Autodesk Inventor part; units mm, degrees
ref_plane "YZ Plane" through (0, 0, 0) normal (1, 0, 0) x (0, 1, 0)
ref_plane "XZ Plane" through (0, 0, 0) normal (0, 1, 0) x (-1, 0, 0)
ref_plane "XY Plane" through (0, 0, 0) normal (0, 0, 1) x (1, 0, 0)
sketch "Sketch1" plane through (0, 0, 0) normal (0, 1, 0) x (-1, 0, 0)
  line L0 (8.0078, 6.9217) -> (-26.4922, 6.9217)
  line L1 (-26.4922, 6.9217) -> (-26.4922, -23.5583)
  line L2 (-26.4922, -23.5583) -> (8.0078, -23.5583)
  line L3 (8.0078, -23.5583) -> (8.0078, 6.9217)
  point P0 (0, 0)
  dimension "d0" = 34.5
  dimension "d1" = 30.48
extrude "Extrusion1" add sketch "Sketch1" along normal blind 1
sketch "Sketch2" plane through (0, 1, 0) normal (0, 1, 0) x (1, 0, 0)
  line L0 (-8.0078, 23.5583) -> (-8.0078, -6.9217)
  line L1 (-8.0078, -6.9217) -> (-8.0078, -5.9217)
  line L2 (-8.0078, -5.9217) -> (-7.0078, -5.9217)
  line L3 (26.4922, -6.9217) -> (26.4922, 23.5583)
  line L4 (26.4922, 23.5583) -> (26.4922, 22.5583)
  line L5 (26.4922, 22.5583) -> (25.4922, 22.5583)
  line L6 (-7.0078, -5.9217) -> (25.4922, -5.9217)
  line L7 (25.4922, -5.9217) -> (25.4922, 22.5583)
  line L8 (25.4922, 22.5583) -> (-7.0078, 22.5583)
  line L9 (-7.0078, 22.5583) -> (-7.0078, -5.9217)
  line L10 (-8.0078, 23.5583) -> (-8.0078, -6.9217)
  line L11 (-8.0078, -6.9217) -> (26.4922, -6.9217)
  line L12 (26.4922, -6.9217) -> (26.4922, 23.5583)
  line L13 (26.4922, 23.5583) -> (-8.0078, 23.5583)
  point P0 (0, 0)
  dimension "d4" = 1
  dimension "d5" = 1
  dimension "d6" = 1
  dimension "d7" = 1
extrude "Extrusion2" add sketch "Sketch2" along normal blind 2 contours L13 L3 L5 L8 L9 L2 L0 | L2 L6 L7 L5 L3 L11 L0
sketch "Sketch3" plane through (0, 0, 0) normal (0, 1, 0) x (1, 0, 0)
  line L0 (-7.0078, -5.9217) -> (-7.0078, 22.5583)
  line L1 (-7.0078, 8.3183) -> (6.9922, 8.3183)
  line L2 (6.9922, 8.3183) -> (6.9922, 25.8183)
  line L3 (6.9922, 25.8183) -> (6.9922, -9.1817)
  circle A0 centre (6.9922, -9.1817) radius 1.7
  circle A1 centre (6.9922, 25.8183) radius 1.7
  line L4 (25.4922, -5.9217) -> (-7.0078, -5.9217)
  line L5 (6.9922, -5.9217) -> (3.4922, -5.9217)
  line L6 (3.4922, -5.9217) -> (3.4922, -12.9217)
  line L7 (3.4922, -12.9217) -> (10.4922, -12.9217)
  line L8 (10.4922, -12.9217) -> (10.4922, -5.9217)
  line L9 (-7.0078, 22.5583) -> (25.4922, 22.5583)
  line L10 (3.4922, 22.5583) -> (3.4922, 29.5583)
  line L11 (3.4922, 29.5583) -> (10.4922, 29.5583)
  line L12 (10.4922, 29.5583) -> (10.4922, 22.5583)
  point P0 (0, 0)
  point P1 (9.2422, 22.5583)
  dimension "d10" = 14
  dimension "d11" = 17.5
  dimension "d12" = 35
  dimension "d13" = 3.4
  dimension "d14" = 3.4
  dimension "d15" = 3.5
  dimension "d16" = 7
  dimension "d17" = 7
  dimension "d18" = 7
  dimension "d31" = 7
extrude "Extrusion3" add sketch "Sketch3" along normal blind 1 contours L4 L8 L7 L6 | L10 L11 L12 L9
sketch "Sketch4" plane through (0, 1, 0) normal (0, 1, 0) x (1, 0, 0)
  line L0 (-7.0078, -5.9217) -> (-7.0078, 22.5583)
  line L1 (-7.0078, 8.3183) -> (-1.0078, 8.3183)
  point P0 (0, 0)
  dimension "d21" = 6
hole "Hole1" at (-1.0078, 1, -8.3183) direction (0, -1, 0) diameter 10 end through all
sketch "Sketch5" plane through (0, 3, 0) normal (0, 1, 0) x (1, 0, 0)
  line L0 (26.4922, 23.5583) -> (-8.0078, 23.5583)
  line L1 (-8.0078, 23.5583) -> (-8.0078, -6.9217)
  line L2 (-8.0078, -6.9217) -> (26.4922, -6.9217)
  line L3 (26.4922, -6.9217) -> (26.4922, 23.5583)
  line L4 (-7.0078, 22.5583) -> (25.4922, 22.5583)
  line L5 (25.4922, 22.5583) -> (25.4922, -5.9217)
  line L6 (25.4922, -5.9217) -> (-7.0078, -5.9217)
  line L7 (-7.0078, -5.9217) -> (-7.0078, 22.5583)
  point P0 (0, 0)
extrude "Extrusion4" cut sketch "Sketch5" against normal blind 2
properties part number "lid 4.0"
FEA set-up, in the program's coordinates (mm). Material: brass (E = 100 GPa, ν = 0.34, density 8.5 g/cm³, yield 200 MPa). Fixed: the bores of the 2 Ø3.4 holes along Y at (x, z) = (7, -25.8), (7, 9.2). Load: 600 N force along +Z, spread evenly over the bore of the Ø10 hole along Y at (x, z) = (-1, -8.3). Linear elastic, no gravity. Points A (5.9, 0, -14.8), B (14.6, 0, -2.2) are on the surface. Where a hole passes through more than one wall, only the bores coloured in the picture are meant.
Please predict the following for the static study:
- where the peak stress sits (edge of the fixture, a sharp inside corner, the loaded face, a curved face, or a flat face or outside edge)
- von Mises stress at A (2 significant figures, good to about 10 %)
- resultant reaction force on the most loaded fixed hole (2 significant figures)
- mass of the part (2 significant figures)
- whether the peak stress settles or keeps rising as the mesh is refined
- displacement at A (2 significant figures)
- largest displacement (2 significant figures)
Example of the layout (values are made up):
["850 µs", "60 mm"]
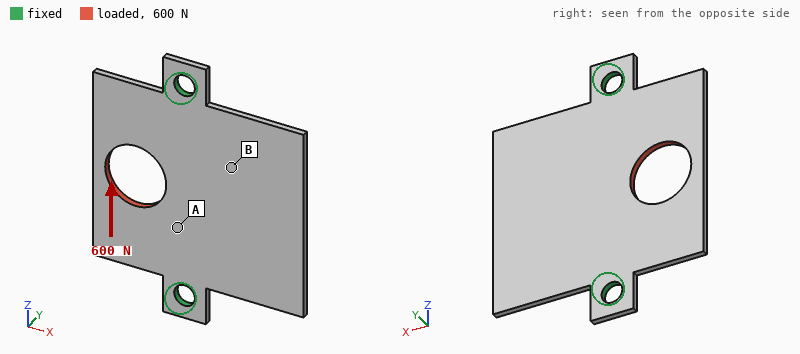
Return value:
["a sharp inside corner", "27 MPa", "330 N", "8.8 g", "keeps rising", "2.9 µm", "14 µm"]
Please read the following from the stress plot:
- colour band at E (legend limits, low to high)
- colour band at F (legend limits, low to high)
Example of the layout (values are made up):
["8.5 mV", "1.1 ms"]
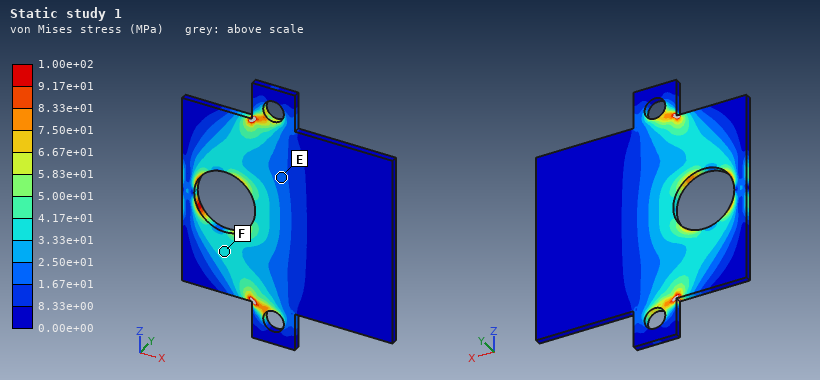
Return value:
["1.67e+01 to 2.50e+01 MPa", "3.33e+01 to 4.17e+01 MPa"]
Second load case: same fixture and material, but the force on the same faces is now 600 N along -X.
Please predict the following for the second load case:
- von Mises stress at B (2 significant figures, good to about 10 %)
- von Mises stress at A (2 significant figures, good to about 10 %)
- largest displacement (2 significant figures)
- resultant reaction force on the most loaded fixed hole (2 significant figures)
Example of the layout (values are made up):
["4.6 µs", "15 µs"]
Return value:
["18 MPa", "16 MPa", "15 µm", "300 N"]
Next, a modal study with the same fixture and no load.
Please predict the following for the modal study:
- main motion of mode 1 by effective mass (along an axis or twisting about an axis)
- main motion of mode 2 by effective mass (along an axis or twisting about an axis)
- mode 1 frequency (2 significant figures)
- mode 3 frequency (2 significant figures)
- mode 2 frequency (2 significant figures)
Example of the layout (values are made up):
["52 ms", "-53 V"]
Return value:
["along Y", "along Y", "1000 Hz", "2600 Hz", "1800 Hz"]
